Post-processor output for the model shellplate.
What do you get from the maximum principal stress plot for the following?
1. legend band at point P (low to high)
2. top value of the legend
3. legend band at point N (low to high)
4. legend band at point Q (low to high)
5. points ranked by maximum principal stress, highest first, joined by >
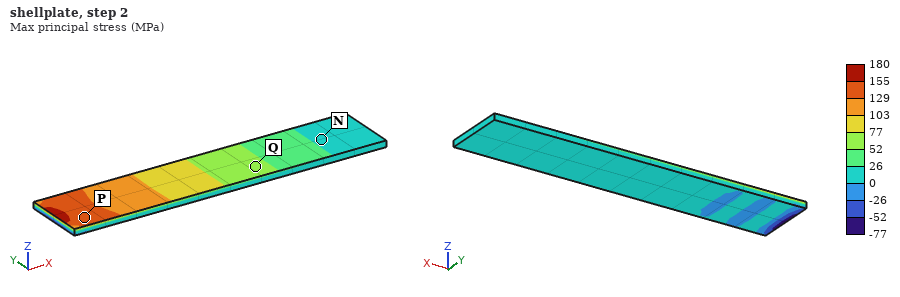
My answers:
129 to 155 MPa
180 MPa
0 to 26 MPa
52 to 77 MPa
P > Q > N
